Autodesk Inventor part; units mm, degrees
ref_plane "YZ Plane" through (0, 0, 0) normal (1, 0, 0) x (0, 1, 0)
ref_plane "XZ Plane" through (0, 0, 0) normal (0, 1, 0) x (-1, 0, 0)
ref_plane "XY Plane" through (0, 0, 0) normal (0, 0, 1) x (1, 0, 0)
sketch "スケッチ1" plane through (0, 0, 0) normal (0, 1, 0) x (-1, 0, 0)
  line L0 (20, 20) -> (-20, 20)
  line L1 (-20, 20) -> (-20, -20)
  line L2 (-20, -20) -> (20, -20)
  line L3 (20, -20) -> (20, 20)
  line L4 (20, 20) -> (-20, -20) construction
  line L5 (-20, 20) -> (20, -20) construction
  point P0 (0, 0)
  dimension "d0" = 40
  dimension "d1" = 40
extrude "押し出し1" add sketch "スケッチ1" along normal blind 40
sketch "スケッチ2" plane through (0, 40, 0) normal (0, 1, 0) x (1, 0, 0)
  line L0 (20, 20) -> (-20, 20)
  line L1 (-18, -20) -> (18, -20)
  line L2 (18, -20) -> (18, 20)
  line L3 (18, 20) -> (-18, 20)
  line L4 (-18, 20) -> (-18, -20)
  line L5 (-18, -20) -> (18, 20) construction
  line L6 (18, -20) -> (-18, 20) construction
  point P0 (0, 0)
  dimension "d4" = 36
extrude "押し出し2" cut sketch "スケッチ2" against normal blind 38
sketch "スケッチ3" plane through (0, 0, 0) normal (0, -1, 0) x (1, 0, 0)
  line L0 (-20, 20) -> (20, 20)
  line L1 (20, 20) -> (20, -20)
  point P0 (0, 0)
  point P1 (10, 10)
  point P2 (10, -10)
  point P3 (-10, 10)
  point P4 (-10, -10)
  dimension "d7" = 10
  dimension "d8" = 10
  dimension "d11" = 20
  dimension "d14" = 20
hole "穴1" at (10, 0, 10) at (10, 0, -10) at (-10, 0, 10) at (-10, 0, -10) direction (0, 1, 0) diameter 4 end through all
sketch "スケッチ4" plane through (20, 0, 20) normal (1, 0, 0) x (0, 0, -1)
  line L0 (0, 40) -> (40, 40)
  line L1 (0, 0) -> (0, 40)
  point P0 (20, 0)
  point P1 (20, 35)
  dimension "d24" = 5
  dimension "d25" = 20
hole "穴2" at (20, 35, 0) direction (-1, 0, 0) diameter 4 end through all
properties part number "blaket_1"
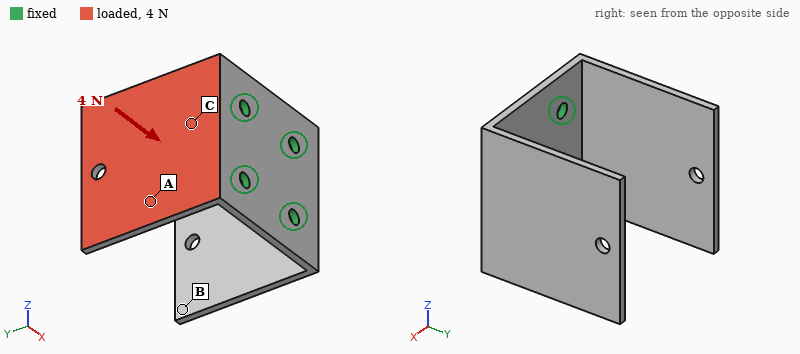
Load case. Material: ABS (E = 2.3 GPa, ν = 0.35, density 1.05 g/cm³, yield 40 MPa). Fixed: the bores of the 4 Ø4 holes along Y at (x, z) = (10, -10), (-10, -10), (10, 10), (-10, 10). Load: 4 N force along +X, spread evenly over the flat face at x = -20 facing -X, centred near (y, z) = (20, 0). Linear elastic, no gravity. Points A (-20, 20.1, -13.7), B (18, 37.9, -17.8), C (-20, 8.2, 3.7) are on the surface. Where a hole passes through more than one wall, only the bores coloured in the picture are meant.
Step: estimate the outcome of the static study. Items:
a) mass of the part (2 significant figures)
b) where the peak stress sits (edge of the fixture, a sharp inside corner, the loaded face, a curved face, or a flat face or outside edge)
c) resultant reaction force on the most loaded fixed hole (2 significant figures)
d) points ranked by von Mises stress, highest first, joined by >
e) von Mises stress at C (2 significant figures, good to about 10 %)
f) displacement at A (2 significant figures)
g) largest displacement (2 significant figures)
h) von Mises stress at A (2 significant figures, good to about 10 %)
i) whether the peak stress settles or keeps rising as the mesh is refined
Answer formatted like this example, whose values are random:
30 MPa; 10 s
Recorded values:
9.6 g; edge of the fixture; 1.8 N; C > A > B; 1.7 MPa; 0.32 mm; 0.78 mm; 0.72 MPa; keeps rising
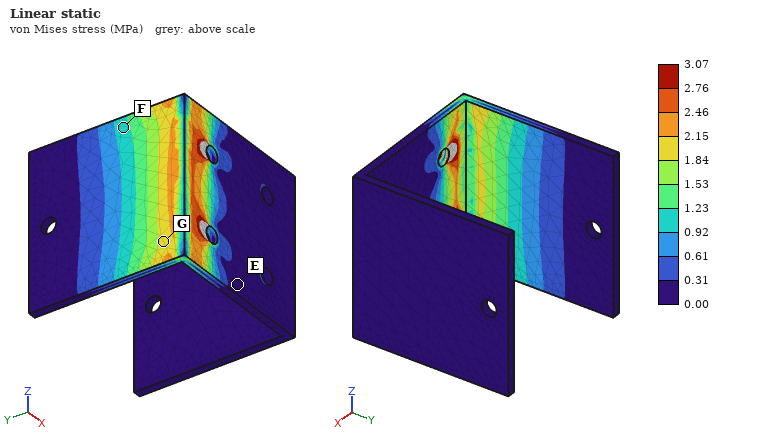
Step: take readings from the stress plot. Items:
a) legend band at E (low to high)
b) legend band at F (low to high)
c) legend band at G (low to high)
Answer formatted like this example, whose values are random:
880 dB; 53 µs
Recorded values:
0.00 to 0.31 MPa; 0.92 to 1.23 MPa; 1.84 to 2.15 MPa
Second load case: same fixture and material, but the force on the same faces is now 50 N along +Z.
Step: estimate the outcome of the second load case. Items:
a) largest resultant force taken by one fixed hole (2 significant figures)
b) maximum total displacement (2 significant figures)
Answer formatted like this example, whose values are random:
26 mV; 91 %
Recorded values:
51 N; 0.74 mm
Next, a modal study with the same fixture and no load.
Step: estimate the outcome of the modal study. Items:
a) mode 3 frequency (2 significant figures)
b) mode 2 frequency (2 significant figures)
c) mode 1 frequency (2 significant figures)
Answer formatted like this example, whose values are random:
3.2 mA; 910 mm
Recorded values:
630 Hz; 250 Hz; 240 Hz
